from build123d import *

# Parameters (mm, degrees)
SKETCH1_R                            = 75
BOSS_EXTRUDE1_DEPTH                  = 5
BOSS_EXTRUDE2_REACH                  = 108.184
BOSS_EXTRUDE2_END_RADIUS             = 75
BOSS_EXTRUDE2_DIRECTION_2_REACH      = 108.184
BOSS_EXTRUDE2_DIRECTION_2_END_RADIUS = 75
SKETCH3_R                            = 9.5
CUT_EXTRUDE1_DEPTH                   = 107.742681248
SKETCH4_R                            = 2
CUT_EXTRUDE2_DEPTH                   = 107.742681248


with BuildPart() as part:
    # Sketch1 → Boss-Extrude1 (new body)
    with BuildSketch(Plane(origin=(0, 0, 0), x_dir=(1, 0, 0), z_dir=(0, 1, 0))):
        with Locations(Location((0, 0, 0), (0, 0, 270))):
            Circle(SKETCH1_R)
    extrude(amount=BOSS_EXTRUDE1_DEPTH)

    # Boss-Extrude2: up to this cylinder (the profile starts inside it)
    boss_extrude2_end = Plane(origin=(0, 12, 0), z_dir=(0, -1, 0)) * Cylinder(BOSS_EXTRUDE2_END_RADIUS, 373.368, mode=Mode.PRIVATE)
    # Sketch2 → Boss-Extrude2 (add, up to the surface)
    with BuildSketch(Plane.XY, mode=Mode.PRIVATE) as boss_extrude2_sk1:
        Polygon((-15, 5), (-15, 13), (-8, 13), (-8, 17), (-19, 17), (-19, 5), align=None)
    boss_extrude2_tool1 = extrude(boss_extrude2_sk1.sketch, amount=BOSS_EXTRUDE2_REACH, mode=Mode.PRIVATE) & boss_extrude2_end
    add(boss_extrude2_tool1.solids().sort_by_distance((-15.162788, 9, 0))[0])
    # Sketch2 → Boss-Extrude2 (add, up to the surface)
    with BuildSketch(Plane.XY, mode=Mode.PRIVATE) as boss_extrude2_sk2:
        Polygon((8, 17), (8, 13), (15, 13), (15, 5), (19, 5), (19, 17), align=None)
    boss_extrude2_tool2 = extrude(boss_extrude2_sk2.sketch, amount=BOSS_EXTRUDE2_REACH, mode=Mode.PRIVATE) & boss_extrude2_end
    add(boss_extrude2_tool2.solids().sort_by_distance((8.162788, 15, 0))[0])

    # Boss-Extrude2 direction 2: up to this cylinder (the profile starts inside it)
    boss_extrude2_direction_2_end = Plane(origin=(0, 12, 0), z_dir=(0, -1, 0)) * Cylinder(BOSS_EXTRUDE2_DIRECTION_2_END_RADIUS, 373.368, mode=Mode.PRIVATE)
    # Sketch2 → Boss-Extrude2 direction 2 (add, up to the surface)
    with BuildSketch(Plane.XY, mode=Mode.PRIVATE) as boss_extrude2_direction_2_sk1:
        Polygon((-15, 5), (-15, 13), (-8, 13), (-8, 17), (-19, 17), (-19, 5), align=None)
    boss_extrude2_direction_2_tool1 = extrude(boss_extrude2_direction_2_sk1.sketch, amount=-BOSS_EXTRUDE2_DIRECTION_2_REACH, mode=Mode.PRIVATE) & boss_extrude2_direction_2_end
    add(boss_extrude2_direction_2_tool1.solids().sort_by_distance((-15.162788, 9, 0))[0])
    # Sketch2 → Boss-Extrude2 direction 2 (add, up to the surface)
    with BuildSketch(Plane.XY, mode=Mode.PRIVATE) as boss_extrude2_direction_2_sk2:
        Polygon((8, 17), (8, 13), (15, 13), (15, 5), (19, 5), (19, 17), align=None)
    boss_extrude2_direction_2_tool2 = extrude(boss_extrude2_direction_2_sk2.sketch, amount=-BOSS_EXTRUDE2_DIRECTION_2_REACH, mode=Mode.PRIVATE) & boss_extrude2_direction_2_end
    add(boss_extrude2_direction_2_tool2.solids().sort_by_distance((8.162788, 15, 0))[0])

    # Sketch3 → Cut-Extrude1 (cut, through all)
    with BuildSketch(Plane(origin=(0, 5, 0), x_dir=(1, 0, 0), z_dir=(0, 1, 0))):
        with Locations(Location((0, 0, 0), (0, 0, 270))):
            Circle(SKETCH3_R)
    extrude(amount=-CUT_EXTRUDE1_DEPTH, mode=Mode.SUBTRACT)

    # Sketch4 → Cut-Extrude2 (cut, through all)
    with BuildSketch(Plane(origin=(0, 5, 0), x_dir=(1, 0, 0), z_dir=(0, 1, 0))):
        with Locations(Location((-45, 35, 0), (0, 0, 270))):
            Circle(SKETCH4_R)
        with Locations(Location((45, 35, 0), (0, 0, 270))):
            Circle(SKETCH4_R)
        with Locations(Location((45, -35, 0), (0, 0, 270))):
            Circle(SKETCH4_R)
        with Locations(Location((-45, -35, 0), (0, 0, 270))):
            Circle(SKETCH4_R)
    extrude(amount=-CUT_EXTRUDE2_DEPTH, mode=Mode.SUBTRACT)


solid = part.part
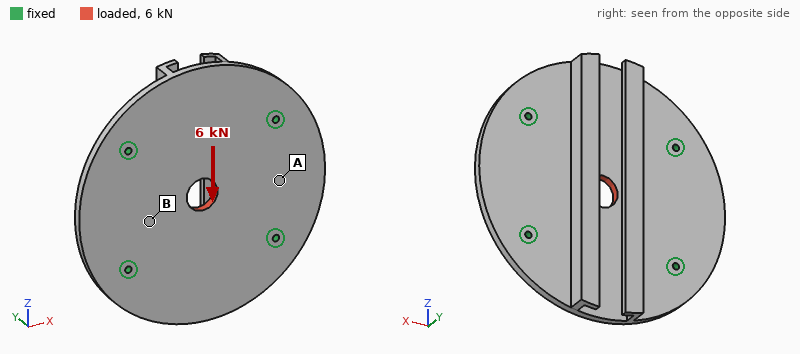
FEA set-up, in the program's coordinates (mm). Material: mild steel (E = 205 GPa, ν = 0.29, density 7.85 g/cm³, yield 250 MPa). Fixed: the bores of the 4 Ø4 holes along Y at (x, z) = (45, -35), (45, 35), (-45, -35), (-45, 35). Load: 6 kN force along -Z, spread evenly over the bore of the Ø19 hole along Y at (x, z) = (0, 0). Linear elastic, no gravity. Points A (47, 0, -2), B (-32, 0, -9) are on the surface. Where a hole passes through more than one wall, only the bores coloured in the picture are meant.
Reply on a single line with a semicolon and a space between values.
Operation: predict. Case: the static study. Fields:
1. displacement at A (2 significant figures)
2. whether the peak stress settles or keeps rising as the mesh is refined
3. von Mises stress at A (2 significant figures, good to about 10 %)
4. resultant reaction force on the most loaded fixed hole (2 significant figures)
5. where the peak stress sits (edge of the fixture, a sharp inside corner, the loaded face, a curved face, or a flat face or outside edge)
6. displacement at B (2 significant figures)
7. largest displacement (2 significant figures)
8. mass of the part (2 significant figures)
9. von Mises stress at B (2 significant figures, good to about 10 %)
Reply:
0.87 µm; keeps rising; 3.2 MPa; 1.5 kN; edge of the fixture; 1.6 µm; 4.4 µm; 860 g; 8.7 MPa
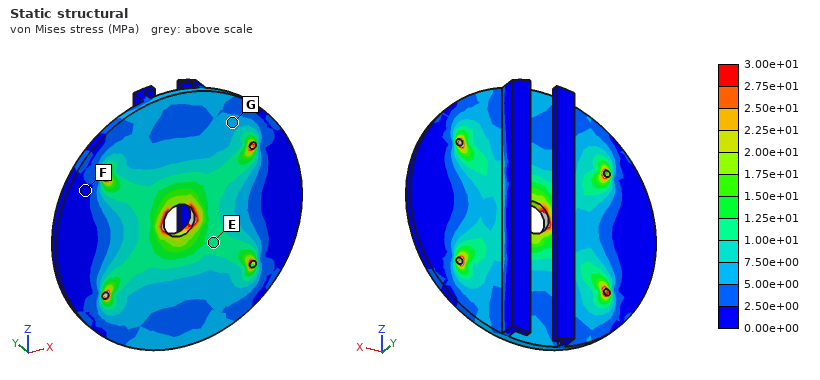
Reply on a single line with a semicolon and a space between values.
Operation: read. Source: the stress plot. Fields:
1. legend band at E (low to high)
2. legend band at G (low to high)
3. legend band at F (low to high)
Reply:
1.00e+01 to 1.25e+01 MPa; 5.00e+00 to 7.50e+00 MPa; 0.00e+00 to 2.50e+00 MPa
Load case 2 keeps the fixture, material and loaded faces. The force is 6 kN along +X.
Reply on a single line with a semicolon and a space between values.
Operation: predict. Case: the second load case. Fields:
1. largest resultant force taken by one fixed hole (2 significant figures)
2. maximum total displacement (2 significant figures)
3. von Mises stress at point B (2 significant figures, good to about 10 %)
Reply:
1.5 kN; 3.8 µm; 8.2 MPa
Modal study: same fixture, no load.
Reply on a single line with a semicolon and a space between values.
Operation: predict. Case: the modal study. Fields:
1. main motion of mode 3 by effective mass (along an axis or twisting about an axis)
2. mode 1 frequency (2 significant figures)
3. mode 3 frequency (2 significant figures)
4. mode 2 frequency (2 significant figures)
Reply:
twisting about Z; 1800 Hz; 3500 Hz; 1800 Hz
